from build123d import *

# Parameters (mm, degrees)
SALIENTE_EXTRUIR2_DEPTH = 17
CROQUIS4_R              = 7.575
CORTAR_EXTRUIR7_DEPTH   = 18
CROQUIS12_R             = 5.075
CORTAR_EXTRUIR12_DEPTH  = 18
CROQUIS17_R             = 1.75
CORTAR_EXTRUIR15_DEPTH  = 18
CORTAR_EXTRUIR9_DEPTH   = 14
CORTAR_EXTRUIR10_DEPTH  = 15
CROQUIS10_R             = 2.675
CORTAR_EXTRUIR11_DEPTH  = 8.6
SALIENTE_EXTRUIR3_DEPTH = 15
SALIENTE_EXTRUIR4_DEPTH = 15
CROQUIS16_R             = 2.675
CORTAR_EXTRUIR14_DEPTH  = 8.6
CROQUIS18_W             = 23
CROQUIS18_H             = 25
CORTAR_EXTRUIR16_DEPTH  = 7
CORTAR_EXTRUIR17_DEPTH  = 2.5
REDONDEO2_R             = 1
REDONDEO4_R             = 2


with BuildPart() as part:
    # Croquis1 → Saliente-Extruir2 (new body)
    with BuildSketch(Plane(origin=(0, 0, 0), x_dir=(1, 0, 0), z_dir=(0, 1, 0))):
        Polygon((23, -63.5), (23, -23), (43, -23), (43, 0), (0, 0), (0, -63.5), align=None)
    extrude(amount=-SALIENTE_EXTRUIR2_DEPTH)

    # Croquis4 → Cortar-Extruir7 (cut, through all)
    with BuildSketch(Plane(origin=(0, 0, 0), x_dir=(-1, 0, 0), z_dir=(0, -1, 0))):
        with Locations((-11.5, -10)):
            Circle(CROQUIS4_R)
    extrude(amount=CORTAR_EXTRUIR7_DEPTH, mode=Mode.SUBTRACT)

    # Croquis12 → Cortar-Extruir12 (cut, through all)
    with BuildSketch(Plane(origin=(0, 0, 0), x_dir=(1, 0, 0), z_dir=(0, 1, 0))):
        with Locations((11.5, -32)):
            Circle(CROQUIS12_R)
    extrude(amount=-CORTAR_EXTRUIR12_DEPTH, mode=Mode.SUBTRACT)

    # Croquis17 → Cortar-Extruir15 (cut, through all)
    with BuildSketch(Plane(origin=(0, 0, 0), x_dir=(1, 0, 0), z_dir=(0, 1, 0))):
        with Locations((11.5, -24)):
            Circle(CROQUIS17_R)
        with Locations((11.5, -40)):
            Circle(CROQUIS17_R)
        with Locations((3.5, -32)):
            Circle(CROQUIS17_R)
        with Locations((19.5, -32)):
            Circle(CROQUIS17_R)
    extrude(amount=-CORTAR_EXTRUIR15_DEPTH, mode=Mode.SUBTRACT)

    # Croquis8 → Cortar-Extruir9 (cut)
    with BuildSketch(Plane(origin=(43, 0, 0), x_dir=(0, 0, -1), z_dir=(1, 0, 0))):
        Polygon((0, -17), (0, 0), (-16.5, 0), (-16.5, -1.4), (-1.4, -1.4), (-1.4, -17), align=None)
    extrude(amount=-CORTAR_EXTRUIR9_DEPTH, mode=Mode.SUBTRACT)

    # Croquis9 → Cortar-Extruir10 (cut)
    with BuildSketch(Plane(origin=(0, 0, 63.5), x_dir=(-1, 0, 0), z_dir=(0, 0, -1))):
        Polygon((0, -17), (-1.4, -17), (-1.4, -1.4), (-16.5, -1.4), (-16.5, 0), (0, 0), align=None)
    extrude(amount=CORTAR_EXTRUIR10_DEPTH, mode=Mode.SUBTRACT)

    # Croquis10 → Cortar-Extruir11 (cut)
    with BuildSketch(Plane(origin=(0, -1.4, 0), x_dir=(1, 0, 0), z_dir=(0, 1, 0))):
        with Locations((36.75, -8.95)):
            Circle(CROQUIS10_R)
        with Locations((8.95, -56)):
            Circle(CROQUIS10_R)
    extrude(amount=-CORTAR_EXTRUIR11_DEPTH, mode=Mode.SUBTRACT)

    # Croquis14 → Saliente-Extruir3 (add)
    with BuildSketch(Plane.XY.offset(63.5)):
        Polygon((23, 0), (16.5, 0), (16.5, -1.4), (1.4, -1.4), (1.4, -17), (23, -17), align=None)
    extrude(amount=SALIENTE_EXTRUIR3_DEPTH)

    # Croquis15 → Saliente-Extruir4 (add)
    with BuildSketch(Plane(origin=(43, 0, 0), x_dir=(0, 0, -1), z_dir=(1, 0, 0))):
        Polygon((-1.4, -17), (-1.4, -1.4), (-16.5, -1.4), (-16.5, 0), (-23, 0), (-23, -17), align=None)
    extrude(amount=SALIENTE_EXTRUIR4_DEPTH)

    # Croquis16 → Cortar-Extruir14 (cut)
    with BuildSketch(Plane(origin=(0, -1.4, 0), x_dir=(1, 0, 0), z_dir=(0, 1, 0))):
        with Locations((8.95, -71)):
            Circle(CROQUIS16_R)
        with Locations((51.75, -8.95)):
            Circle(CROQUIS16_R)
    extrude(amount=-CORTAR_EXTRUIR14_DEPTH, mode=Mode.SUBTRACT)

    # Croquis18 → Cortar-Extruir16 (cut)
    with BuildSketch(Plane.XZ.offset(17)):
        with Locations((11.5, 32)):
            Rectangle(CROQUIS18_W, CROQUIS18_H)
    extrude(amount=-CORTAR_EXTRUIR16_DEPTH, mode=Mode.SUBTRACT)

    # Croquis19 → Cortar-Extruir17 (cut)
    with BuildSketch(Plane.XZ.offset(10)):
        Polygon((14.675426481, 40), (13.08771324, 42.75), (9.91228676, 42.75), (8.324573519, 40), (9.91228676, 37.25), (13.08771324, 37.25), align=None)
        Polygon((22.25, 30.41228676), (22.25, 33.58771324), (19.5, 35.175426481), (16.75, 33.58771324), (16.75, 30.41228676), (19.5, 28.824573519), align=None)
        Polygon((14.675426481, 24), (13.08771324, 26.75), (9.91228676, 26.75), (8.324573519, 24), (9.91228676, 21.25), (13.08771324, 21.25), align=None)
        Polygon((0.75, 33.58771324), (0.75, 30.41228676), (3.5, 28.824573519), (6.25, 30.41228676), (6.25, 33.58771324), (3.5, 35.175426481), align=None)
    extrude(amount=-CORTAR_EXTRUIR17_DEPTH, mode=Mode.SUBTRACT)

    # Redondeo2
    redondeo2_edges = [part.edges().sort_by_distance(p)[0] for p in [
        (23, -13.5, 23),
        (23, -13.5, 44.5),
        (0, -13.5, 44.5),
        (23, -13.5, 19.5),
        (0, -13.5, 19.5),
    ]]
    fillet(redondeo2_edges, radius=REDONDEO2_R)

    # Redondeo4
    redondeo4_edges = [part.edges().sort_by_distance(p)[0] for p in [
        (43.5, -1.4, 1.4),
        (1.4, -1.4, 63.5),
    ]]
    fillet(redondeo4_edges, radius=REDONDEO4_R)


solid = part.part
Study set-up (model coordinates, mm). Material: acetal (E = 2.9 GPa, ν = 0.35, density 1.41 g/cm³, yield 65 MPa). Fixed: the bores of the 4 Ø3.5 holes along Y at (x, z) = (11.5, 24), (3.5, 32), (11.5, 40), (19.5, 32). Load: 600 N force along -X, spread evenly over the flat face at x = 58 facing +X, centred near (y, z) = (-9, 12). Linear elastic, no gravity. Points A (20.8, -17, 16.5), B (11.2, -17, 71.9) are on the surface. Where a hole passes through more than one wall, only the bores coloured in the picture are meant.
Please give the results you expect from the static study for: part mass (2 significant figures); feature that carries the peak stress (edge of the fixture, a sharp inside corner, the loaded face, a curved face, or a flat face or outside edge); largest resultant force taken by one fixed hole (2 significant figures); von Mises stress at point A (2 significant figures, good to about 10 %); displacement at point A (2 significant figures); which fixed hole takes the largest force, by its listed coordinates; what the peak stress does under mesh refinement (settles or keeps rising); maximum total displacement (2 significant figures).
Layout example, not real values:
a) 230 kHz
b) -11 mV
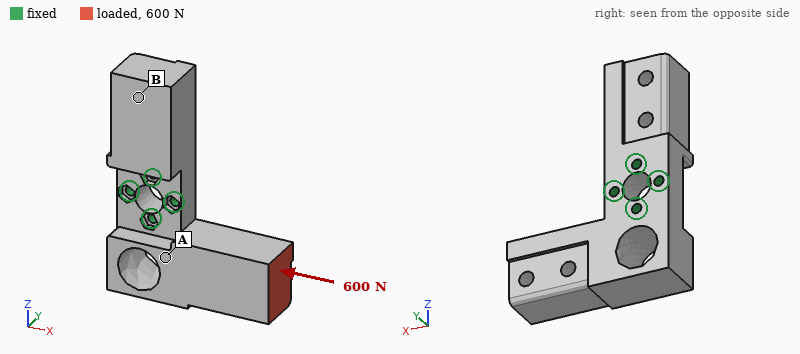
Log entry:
a) 46 g
b) edge of the fixture
c) 670 N
d) 4.6 MPa
e) 0.13 mm
f) (11.5, 24)
g) keeps rising
h) 0.48 mm
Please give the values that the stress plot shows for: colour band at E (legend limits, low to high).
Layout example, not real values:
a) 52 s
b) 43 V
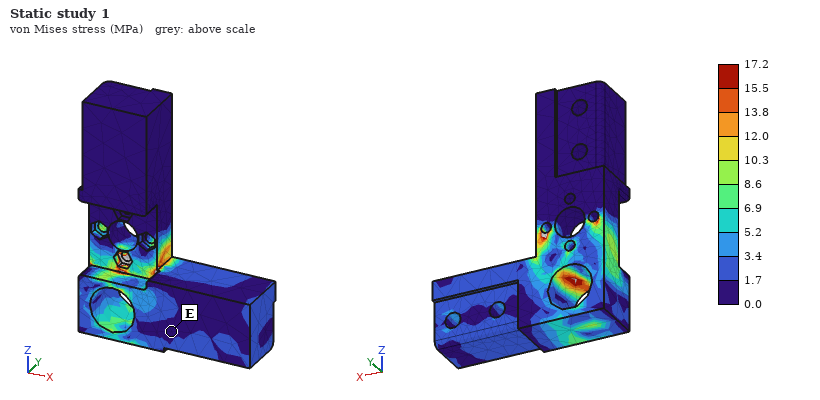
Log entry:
a) 0.0 to 1.7 MPa
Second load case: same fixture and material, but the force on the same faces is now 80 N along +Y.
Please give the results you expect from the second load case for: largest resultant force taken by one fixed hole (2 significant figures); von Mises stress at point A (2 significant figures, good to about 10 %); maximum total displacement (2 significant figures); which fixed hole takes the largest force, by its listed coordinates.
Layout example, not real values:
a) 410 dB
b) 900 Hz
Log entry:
a) 100 N
b) 5.8 MPa
c) 0.60 mm
d) (19.5, 32)
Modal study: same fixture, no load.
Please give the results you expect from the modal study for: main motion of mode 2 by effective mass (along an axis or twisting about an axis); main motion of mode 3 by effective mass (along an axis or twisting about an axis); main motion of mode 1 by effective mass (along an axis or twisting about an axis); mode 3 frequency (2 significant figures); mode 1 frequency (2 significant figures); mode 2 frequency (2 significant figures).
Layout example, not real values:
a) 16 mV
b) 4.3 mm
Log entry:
a) along Z
b) along Y
c) along Y
d) 1100 Hz
e) 700 Hz
f) 1000 Hz
